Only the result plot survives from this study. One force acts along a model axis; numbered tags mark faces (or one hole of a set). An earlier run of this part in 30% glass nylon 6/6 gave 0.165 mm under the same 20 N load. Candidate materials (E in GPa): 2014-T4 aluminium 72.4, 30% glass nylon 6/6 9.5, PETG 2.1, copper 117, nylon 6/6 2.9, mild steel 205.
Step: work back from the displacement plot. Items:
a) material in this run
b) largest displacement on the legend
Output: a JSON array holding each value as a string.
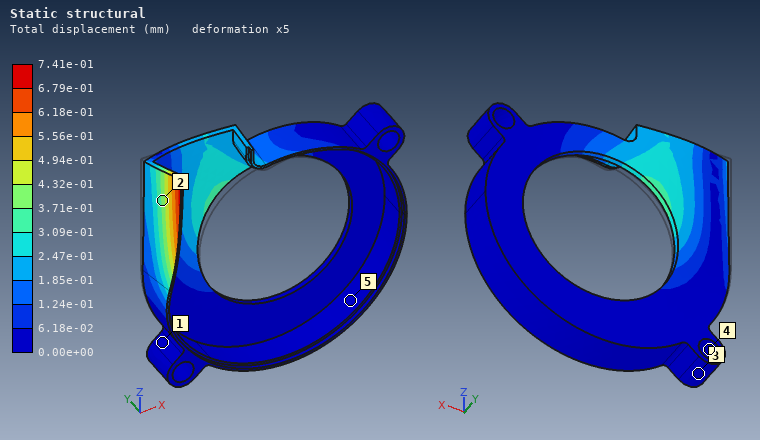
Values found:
["PETG", "7.41e-01 mm"]
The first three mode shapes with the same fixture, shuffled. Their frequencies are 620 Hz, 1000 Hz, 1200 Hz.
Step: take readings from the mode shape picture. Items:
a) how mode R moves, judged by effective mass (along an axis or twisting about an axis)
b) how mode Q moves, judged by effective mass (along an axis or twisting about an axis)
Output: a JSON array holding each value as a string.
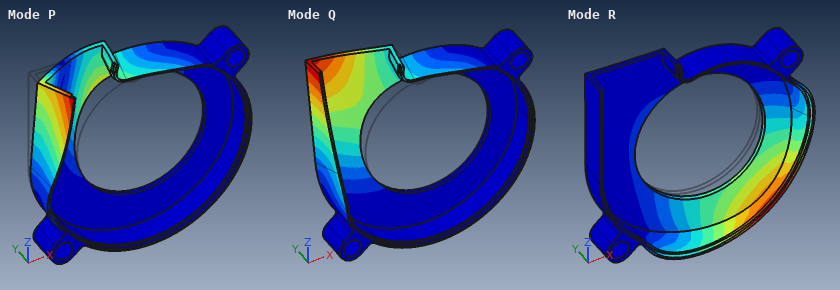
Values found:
["along Y", "along Y"]
